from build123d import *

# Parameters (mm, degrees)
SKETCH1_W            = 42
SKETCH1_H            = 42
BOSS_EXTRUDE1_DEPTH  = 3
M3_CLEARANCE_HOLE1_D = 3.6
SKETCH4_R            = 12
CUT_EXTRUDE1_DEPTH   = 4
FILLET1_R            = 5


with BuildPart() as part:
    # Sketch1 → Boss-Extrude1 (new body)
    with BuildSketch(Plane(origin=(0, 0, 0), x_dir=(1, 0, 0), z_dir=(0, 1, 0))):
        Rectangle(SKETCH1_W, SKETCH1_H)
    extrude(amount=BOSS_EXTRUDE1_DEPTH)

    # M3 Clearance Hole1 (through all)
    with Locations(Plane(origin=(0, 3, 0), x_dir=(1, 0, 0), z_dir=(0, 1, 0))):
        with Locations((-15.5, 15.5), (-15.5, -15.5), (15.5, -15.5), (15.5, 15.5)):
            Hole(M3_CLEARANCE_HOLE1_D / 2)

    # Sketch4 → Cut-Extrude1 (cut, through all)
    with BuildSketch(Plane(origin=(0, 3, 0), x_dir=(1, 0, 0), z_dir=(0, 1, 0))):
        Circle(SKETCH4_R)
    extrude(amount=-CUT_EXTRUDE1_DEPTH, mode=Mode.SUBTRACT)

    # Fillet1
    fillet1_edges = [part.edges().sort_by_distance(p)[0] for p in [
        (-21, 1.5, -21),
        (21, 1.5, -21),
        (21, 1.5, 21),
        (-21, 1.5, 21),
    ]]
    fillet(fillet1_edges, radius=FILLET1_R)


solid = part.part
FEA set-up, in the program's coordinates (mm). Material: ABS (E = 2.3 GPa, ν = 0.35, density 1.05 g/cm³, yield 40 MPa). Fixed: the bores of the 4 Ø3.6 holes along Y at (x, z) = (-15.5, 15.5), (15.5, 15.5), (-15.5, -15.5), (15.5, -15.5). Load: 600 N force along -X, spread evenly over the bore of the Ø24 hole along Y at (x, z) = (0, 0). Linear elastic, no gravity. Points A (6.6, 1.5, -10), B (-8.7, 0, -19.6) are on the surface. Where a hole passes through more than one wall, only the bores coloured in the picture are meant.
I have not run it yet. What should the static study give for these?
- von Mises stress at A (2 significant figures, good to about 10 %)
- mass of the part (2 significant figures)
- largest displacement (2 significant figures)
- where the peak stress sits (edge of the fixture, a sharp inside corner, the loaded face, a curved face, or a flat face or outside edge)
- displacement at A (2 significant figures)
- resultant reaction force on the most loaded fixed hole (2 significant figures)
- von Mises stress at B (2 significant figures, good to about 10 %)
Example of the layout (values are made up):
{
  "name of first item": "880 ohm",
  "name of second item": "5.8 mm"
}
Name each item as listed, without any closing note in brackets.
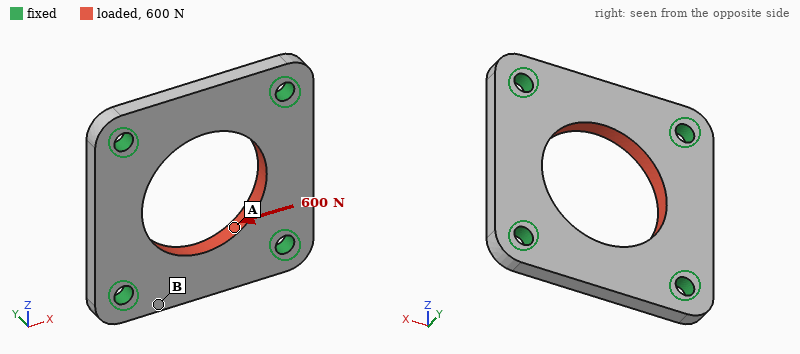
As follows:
{
  "von Mises stress at A": "6.7 MPa",
  "mass of the part": "3.9 g",
  "largest displacement": "59 µm",
  "where the peak stress sits": "edge of the fixture",
  "displacement at A": "28 µm",
  "resultant reaction force on the most loaded fixed hole": "150 N",
  "von Mises stress at B": "2.7 MPa"
}
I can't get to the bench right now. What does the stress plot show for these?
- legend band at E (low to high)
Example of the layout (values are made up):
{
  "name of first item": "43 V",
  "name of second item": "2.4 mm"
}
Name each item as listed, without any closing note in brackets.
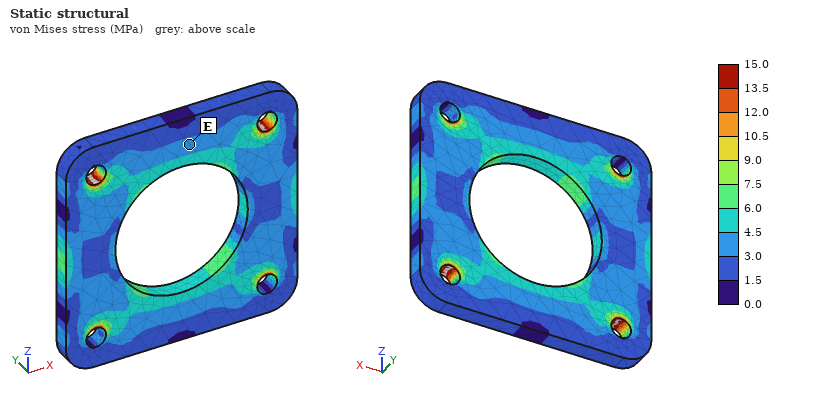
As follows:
{
  "legend band at E": "3.0 to 4.5 MPa"
}
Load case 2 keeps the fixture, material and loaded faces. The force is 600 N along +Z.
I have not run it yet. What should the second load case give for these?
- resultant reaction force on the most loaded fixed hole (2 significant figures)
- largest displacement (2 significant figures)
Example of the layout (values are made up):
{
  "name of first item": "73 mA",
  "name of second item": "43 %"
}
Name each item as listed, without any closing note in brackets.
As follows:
{
  "resultant reaction force on the most loaded fixed hole": "150 N",
  "largest displacement": "59 µm"
}
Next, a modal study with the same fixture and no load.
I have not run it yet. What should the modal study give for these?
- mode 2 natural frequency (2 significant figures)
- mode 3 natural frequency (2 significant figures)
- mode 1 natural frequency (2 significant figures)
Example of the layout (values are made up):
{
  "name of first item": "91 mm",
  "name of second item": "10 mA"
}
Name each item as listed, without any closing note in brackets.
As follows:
{
  "mode 2 natural frequency": "5200 Hz",
  "mode 3 natural frequency": "5300 Hz",
  "mode 1 natural frequency": "5100 Hz"
}
